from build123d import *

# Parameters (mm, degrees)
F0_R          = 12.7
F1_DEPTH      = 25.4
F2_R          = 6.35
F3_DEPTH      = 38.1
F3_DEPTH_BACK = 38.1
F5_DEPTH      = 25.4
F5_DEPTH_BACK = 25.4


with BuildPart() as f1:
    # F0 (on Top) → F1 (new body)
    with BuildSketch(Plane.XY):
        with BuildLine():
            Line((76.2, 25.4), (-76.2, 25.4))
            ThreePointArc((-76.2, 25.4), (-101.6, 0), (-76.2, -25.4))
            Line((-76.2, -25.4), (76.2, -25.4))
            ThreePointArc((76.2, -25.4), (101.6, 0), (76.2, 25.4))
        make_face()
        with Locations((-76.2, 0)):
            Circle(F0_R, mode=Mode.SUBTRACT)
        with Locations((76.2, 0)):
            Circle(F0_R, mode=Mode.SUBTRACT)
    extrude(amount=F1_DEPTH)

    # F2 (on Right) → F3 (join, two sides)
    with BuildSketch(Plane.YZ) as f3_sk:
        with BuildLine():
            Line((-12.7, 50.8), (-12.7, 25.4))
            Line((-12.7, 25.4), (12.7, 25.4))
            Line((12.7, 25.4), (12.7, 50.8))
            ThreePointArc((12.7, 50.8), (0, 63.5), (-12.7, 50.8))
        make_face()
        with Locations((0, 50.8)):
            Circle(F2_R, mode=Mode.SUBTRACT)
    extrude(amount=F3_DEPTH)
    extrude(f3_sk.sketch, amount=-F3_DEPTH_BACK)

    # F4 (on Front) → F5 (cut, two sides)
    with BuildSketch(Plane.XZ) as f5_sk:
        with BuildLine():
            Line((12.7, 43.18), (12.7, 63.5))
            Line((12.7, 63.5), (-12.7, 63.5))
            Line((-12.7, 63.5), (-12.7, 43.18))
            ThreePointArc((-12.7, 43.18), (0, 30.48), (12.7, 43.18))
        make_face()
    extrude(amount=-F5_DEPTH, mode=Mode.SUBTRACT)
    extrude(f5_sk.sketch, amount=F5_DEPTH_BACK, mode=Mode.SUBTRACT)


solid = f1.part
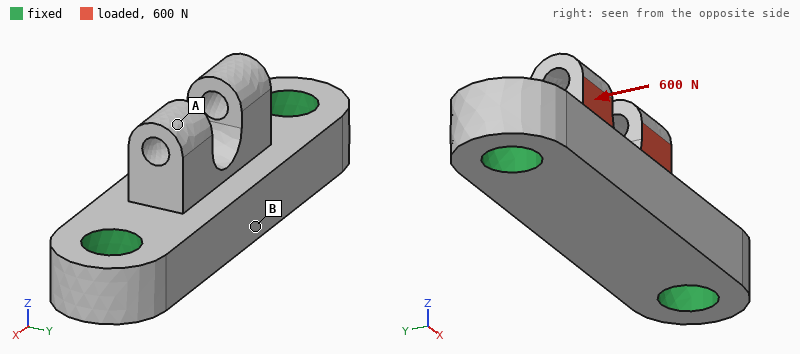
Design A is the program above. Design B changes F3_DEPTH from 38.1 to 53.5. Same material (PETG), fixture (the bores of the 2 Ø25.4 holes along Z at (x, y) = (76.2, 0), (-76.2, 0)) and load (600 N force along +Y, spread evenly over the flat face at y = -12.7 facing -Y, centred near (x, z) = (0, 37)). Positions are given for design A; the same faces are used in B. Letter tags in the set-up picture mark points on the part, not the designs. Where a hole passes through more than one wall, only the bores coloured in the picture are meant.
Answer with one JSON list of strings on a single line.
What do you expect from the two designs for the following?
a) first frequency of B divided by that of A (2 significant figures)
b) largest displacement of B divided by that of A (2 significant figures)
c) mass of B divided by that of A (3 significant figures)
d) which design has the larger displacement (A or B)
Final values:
["1.0", "0.83", "1.04", "A"]
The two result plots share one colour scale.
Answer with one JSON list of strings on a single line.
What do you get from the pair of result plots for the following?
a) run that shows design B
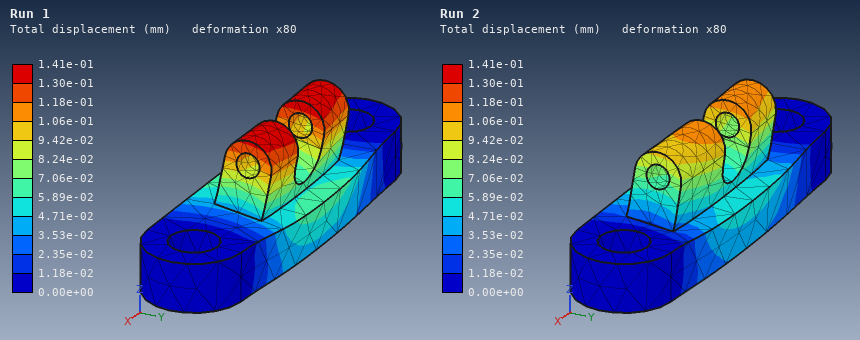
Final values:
["Run 2"]
